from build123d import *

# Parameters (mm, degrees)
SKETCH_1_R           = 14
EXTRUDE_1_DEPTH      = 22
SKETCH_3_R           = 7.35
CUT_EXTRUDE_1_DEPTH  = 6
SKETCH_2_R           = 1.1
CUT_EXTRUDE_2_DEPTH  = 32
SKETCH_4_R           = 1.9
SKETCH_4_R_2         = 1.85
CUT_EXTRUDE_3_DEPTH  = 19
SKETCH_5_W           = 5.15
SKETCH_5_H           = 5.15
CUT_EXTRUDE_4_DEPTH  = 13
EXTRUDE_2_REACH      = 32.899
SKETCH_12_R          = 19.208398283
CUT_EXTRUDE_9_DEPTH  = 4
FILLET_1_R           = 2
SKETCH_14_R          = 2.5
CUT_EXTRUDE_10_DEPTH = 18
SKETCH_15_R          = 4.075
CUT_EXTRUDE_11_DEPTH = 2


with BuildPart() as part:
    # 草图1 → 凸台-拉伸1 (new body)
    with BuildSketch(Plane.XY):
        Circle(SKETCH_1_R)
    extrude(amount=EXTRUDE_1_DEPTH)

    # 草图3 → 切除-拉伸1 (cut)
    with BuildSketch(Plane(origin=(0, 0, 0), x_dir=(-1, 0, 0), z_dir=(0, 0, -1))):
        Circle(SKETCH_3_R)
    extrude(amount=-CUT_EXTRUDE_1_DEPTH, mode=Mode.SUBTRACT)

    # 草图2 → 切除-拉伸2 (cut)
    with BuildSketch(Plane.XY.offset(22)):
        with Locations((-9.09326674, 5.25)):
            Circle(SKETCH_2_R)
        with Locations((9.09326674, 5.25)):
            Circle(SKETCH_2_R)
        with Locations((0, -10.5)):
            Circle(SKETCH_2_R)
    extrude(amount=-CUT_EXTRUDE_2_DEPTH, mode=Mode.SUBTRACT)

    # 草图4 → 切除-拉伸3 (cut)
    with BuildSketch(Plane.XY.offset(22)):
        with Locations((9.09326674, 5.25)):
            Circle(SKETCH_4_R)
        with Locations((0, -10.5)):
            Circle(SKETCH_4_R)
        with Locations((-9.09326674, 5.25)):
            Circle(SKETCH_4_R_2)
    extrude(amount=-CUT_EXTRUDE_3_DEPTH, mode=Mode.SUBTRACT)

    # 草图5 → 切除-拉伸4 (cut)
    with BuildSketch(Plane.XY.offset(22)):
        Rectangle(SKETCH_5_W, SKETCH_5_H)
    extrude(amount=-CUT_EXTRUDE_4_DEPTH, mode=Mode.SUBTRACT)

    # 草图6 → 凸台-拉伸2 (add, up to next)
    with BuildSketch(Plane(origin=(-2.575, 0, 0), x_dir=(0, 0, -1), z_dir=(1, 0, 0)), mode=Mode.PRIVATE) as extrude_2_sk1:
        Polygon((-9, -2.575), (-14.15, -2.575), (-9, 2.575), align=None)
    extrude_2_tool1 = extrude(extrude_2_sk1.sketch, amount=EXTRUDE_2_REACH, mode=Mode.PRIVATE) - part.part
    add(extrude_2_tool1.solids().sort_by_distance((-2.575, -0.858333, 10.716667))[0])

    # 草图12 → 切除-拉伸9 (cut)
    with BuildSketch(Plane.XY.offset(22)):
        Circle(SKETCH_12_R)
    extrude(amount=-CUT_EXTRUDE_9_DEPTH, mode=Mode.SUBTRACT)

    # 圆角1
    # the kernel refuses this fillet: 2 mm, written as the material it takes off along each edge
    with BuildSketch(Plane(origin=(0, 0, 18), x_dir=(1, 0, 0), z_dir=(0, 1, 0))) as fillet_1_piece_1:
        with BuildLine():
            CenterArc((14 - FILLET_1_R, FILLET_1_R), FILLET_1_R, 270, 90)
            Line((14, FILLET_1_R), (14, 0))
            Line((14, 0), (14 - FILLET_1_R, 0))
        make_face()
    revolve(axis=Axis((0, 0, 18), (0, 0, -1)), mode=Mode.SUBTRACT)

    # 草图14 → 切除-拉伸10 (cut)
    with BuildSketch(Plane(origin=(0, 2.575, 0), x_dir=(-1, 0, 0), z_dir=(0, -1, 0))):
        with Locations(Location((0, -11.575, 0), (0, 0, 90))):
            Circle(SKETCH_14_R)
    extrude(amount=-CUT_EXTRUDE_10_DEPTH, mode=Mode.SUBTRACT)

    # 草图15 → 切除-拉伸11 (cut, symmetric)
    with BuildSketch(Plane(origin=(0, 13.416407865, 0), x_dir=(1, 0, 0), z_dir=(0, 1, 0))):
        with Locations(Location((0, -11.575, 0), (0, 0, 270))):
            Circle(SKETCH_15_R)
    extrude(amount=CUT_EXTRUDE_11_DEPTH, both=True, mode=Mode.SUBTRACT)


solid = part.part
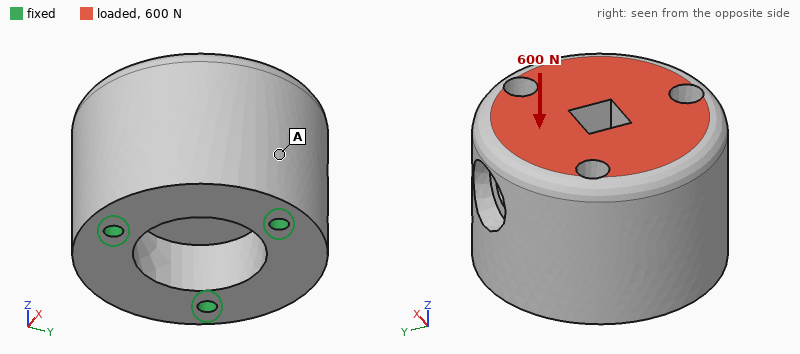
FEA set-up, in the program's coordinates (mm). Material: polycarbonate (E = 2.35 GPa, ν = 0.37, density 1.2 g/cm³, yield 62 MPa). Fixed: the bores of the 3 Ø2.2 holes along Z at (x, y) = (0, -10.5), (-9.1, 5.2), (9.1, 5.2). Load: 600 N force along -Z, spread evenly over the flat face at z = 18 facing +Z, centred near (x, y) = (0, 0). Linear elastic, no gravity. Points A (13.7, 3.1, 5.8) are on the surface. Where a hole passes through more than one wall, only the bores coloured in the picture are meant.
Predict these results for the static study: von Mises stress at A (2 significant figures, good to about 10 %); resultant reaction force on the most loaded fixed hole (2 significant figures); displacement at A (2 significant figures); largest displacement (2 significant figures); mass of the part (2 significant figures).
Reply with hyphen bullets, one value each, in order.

- 2.2 MPa
- 200 N
- 21 µm
- 36 µm
- 11 g
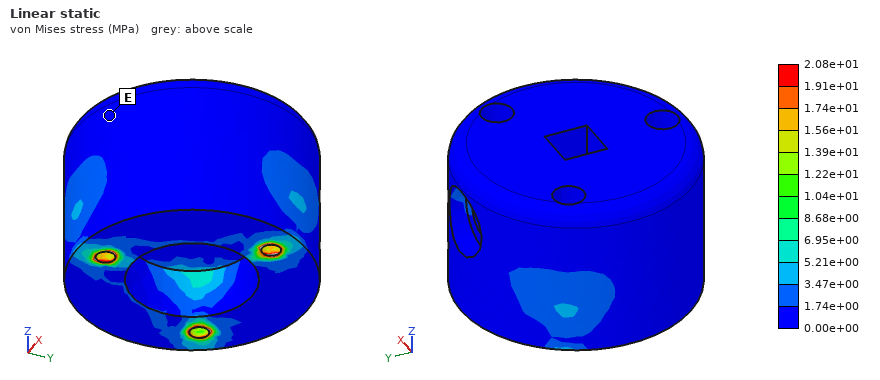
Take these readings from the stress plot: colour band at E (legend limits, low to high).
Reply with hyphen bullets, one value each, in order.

- 0.00e+00 to 1.74e+00 MPa
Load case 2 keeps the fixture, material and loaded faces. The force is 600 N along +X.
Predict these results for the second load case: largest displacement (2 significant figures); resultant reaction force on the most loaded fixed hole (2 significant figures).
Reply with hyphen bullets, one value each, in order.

- 0.20 mm
- 530 N
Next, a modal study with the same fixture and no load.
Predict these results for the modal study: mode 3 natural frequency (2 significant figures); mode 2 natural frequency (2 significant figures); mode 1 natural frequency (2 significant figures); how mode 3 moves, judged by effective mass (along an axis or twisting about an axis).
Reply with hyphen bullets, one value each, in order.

- 7700 Hz
- 4400 Hz
- 4300 Hz
- along Z
